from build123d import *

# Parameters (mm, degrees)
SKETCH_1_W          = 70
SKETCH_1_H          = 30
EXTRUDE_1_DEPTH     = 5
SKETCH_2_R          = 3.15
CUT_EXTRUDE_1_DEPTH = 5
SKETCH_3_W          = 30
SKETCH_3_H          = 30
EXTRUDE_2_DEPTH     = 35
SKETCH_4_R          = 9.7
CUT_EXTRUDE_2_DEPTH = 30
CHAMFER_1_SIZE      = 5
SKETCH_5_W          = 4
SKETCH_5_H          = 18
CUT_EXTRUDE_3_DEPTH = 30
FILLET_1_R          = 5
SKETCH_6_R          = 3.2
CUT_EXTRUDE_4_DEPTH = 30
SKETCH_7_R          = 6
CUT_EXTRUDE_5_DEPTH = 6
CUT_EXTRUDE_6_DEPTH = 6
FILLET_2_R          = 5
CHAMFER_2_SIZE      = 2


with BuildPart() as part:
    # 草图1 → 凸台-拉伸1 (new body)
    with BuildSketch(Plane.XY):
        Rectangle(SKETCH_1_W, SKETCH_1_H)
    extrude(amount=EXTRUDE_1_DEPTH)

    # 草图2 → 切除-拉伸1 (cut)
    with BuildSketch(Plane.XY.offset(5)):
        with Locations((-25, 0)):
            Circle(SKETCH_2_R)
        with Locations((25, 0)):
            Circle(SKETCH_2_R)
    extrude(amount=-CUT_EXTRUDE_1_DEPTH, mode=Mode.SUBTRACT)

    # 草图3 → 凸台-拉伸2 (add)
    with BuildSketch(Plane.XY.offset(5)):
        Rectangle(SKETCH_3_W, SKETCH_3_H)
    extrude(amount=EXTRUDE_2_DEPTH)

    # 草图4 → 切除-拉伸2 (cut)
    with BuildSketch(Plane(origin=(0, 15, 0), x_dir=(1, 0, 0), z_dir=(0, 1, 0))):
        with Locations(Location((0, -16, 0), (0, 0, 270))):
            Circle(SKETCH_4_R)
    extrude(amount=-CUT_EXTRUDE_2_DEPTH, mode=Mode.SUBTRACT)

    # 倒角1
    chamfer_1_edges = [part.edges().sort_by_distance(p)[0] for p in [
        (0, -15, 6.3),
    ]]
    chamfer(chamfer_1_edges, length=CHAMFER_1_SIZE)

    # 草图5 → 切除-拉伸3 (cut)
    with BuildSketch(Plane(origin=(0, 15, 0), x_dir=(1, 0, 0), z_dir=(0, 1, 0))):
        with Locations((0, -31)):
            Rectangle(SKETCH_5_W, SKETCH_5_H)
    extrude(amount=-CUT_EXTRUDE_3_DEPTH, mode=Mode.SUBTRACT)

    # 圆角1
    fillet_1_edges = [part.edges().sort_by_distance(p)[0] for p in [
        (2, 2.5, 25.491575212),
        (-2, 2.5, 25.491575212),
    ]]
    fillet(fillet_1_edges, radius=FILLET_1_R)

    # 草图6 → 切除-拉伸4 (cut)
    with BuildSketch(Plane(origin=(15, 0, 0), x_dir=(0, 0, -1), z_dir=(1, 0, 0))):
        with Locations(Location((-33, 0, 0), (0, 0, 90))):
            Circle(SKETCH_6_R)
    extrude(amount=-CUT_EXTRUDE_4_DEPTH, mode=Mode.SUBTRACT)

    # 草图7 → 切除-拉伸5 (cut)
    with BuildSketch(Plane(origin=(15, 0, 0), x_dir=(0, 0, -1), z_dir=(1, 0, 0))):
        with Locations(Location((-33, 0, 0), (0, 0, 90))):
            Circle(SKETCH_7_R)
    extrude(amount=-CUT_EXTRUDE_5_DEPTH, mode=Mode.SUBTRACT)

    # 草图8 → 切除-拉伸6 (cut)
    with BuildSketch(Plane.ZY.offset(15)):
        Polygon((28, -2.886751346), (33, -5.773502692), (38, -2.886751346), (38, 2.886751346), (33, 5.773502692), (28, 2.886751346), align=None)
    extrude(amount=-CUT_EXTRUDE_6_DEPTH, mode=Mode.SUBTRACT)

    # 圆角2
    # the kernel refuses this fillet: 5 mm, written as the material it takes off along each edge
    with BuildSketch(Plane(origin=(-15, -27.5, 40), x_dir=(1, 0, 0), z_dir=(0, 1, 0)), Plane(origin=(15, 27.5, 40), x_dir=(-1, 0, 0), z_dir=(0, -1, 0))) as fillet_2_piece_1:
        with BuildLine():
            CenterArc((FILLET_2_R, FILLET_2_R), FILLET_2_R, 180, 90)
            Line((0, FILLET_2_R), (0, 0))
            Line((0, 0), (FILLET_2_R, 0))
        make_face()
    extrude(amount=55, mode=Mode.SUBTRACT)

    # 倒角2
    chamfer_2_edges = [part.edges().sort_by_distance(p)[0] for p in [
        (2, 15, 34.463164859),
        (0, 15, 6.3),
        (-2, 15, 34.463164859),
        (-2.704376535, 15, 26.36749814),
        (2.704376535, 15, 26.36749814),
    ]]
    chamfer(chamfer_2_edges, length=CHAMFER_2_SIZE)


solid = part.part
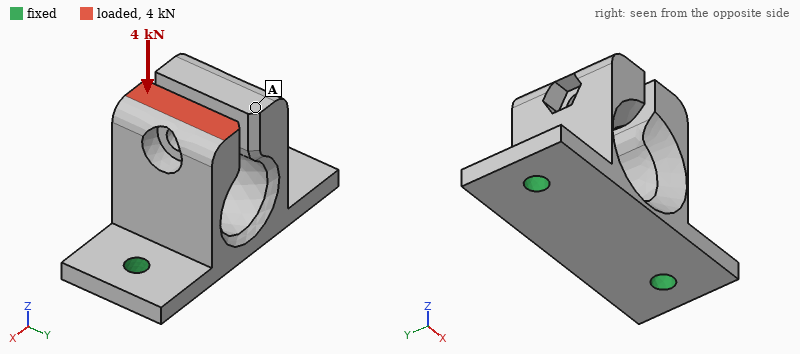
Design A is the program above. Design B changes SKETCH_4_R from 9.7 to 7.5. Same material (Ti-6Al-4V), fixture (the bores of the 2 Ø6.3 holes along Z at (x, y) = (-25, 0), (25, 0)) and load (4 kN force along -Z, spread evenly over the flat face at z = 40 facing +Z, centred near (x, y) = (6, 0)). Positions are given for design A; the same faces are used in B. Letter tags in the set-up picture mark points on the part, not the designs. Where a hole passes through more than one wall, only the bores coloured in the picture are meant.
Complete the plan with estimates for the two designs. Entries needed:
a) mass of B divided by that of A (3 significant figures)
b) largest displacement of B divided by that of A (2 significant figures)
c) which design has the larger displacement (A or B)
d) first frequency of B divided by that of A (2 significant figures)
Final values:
1.13
0.35
A
0.97
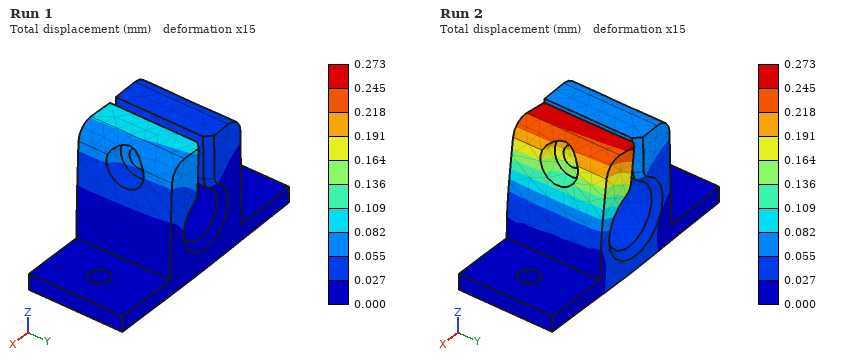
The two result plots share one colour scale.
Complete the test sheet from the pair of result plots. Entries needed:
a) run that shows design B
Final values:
Run 1
